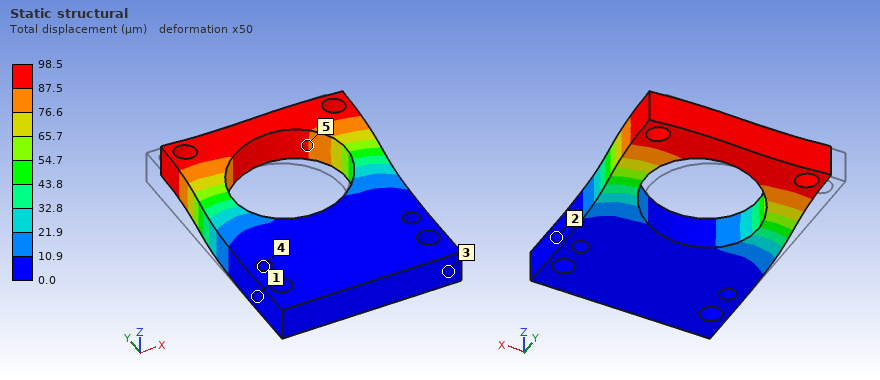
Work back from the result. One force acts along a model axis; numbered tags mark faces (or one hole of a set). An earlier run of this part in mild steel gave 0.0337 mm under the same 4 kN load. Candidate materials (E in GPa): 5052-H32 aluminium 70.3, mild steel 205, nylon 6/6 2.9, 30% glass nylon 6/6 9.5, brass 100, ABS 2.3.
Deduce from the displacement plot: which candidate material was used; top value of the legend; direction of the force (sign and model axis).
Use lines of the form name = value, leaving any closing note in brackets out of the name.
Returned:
which candidate material was used = 5052-H32 aluminium
top value of the legend = 98.5 µm
direction of the force = +X
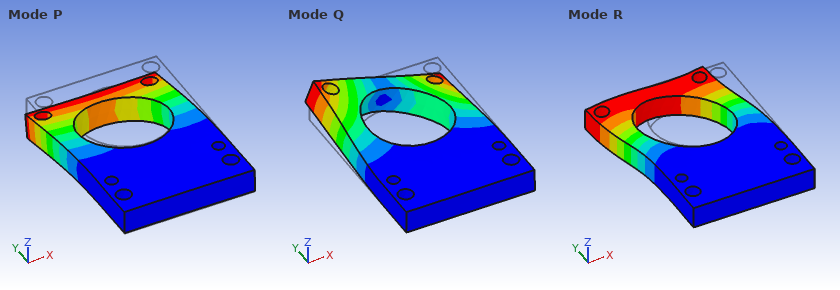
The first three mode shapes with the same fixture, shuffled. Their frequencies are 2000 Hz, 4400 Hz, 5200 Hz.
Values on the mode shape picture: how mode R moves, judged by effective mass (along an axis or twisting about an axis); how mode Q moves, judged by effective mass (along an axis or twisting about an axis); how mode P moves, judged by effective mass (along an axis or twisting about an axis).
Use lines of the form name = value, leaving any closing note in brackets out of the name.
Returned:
how mode R moves, judged by effective mass = along X
how mode Q moves, judged by effective mass = twisting about Y
how mode P moves, judged by effective mass = along Z
